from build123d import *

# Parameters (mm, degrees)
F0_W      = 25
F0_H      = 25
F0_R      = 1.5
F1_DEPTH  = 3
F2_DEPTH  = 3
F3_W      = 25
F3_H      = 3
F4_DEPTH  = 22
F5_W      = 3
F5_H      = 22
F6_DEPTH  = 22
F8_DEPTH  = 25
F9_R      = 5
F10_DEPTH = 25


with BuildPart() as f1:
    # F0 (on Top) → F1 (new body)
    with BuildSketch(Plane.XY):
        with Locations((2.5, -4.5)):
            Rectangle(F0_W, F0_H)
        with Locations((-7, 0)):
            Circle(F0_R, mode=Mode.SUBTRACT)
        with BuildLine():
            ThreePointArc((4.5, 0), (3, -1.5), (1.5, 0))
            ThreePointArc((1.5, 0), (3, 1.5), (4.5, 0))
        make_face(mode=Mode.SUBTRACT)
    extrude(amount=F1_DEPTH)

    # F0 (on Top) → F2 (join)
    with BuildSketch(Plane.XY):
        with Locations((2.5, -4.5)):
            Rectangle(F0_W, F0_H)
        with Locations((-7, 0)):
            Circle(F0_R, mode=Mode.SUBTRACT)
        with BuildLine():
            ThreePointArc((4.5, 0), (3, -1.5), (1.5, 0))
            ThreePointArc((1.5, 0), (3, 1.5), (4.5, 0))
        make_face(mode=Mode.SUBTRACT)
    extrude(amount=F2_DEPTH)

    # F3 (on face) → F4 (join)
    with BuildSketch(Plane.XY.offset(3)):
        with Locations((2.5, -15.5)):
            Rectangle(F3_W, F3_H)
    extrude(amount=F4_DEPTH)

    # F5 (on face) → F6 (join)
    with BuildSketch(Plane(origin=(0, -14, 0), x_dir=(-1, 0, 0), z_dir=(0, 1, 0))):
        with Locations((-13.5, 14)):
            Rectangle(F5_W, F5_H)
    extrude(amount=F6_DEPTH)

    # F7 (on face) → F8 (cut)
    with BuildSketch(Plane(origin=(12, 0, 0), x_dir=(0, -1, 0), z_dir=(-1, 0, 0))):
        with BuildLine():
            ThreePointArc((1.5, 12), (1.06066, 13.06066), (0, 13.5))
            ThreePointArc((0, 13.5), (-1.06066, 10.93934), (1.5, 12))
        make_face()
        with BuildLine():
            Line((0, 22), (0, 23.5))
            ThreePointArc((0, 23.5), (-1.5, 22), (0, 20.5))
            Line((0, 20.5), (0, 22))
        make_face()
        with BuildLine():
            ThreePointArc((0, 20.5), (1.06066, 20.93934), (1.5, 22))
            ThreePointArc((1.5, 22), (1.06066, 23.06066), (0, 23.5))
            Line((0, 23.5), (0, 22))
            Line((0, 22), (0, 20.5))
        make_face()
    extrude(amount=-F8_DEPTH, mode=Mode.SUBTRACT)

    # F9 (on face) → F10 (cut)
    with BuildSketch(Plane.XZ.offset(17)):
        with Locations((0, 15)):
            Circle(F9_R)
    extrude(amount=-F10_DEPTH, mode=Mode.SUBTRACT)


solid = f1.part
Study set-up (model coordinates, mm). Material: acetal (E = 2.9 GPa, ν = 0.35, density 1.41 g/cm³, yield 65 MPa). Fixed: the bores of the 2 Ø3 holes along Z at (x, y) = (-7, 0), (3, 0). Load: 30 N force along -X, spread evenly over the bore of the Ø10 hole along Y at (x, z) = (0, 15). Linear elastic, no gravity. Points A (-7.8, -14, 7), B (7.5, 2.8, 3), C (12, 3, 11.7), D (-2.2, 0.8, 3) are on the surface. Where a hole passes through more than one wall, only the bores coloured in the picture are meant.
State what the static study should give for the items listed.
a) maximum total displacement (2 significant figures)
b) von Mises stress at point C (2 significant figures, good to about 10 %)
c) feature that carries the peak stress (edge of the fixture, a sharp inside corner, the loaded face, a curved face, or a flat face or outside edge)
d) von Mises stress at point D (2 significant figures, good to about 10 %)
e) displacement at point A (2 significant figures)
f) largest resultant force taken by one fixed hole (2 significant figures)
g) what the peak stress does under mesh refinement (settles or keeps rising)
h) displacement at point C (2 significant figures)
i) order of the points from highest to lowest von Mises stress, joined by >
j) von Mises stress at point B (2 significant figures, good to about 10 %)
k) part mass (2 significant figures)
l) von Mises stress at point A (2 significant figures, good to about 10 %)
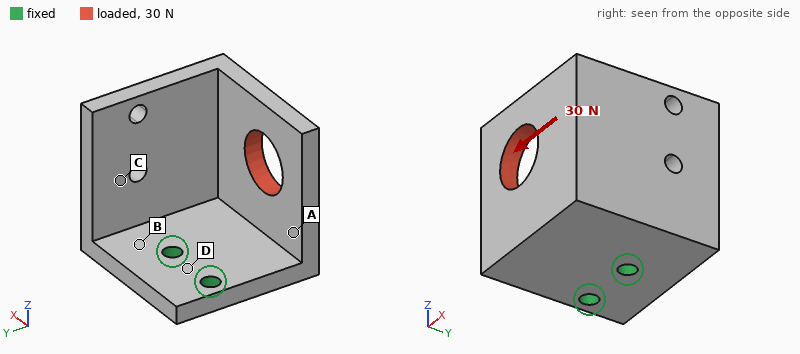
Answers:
0.41 mm
1.0 MPa
edge of the fixture
1.9 MPa
0.14 mm
49 N
keeps rising
0.13 mm
B > A > D > C
5.2 MPa
6.6 g
3.9 MPa
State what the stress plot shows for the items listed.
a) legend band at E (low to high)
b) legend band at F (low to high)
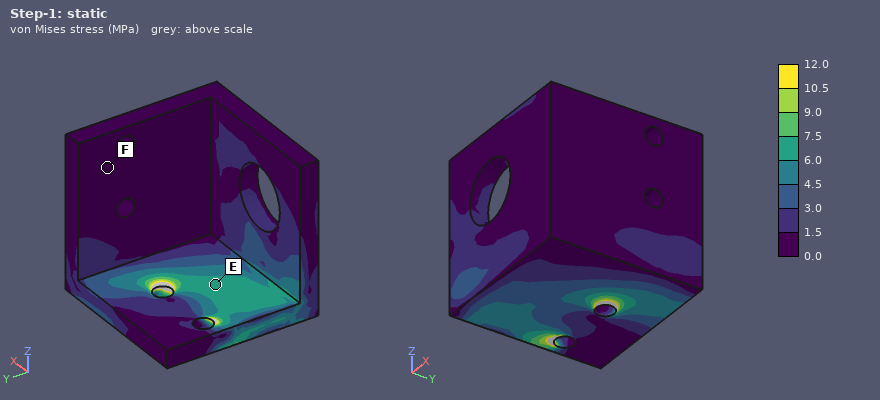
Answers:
6.0 to 7.5 MPa
0.0 to 1.5 MPa
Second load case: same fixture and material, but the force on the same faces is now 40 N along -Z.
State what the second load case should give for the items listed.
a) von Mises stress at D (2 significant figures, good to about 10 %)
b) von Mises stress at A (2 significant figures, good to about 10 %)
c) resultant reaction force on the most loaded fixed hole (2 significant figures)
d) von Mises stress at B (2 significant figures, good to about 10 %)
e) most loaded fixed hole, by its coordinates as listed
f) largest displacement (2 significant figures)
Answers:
3.3 MPa
2.6 MPa
25 N
6.4 MPa
(3, 0)
0.51 mm
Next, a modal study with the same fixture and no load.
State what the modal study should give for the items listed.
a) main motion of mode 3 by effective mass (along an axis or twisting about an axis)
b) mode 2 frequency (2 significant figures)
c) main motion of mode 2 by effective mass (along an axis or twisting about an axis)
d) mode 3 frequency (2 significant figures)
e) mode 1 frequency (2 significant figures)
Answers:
along Z
890 Hz
along X
2000 Hz
670 Hz
